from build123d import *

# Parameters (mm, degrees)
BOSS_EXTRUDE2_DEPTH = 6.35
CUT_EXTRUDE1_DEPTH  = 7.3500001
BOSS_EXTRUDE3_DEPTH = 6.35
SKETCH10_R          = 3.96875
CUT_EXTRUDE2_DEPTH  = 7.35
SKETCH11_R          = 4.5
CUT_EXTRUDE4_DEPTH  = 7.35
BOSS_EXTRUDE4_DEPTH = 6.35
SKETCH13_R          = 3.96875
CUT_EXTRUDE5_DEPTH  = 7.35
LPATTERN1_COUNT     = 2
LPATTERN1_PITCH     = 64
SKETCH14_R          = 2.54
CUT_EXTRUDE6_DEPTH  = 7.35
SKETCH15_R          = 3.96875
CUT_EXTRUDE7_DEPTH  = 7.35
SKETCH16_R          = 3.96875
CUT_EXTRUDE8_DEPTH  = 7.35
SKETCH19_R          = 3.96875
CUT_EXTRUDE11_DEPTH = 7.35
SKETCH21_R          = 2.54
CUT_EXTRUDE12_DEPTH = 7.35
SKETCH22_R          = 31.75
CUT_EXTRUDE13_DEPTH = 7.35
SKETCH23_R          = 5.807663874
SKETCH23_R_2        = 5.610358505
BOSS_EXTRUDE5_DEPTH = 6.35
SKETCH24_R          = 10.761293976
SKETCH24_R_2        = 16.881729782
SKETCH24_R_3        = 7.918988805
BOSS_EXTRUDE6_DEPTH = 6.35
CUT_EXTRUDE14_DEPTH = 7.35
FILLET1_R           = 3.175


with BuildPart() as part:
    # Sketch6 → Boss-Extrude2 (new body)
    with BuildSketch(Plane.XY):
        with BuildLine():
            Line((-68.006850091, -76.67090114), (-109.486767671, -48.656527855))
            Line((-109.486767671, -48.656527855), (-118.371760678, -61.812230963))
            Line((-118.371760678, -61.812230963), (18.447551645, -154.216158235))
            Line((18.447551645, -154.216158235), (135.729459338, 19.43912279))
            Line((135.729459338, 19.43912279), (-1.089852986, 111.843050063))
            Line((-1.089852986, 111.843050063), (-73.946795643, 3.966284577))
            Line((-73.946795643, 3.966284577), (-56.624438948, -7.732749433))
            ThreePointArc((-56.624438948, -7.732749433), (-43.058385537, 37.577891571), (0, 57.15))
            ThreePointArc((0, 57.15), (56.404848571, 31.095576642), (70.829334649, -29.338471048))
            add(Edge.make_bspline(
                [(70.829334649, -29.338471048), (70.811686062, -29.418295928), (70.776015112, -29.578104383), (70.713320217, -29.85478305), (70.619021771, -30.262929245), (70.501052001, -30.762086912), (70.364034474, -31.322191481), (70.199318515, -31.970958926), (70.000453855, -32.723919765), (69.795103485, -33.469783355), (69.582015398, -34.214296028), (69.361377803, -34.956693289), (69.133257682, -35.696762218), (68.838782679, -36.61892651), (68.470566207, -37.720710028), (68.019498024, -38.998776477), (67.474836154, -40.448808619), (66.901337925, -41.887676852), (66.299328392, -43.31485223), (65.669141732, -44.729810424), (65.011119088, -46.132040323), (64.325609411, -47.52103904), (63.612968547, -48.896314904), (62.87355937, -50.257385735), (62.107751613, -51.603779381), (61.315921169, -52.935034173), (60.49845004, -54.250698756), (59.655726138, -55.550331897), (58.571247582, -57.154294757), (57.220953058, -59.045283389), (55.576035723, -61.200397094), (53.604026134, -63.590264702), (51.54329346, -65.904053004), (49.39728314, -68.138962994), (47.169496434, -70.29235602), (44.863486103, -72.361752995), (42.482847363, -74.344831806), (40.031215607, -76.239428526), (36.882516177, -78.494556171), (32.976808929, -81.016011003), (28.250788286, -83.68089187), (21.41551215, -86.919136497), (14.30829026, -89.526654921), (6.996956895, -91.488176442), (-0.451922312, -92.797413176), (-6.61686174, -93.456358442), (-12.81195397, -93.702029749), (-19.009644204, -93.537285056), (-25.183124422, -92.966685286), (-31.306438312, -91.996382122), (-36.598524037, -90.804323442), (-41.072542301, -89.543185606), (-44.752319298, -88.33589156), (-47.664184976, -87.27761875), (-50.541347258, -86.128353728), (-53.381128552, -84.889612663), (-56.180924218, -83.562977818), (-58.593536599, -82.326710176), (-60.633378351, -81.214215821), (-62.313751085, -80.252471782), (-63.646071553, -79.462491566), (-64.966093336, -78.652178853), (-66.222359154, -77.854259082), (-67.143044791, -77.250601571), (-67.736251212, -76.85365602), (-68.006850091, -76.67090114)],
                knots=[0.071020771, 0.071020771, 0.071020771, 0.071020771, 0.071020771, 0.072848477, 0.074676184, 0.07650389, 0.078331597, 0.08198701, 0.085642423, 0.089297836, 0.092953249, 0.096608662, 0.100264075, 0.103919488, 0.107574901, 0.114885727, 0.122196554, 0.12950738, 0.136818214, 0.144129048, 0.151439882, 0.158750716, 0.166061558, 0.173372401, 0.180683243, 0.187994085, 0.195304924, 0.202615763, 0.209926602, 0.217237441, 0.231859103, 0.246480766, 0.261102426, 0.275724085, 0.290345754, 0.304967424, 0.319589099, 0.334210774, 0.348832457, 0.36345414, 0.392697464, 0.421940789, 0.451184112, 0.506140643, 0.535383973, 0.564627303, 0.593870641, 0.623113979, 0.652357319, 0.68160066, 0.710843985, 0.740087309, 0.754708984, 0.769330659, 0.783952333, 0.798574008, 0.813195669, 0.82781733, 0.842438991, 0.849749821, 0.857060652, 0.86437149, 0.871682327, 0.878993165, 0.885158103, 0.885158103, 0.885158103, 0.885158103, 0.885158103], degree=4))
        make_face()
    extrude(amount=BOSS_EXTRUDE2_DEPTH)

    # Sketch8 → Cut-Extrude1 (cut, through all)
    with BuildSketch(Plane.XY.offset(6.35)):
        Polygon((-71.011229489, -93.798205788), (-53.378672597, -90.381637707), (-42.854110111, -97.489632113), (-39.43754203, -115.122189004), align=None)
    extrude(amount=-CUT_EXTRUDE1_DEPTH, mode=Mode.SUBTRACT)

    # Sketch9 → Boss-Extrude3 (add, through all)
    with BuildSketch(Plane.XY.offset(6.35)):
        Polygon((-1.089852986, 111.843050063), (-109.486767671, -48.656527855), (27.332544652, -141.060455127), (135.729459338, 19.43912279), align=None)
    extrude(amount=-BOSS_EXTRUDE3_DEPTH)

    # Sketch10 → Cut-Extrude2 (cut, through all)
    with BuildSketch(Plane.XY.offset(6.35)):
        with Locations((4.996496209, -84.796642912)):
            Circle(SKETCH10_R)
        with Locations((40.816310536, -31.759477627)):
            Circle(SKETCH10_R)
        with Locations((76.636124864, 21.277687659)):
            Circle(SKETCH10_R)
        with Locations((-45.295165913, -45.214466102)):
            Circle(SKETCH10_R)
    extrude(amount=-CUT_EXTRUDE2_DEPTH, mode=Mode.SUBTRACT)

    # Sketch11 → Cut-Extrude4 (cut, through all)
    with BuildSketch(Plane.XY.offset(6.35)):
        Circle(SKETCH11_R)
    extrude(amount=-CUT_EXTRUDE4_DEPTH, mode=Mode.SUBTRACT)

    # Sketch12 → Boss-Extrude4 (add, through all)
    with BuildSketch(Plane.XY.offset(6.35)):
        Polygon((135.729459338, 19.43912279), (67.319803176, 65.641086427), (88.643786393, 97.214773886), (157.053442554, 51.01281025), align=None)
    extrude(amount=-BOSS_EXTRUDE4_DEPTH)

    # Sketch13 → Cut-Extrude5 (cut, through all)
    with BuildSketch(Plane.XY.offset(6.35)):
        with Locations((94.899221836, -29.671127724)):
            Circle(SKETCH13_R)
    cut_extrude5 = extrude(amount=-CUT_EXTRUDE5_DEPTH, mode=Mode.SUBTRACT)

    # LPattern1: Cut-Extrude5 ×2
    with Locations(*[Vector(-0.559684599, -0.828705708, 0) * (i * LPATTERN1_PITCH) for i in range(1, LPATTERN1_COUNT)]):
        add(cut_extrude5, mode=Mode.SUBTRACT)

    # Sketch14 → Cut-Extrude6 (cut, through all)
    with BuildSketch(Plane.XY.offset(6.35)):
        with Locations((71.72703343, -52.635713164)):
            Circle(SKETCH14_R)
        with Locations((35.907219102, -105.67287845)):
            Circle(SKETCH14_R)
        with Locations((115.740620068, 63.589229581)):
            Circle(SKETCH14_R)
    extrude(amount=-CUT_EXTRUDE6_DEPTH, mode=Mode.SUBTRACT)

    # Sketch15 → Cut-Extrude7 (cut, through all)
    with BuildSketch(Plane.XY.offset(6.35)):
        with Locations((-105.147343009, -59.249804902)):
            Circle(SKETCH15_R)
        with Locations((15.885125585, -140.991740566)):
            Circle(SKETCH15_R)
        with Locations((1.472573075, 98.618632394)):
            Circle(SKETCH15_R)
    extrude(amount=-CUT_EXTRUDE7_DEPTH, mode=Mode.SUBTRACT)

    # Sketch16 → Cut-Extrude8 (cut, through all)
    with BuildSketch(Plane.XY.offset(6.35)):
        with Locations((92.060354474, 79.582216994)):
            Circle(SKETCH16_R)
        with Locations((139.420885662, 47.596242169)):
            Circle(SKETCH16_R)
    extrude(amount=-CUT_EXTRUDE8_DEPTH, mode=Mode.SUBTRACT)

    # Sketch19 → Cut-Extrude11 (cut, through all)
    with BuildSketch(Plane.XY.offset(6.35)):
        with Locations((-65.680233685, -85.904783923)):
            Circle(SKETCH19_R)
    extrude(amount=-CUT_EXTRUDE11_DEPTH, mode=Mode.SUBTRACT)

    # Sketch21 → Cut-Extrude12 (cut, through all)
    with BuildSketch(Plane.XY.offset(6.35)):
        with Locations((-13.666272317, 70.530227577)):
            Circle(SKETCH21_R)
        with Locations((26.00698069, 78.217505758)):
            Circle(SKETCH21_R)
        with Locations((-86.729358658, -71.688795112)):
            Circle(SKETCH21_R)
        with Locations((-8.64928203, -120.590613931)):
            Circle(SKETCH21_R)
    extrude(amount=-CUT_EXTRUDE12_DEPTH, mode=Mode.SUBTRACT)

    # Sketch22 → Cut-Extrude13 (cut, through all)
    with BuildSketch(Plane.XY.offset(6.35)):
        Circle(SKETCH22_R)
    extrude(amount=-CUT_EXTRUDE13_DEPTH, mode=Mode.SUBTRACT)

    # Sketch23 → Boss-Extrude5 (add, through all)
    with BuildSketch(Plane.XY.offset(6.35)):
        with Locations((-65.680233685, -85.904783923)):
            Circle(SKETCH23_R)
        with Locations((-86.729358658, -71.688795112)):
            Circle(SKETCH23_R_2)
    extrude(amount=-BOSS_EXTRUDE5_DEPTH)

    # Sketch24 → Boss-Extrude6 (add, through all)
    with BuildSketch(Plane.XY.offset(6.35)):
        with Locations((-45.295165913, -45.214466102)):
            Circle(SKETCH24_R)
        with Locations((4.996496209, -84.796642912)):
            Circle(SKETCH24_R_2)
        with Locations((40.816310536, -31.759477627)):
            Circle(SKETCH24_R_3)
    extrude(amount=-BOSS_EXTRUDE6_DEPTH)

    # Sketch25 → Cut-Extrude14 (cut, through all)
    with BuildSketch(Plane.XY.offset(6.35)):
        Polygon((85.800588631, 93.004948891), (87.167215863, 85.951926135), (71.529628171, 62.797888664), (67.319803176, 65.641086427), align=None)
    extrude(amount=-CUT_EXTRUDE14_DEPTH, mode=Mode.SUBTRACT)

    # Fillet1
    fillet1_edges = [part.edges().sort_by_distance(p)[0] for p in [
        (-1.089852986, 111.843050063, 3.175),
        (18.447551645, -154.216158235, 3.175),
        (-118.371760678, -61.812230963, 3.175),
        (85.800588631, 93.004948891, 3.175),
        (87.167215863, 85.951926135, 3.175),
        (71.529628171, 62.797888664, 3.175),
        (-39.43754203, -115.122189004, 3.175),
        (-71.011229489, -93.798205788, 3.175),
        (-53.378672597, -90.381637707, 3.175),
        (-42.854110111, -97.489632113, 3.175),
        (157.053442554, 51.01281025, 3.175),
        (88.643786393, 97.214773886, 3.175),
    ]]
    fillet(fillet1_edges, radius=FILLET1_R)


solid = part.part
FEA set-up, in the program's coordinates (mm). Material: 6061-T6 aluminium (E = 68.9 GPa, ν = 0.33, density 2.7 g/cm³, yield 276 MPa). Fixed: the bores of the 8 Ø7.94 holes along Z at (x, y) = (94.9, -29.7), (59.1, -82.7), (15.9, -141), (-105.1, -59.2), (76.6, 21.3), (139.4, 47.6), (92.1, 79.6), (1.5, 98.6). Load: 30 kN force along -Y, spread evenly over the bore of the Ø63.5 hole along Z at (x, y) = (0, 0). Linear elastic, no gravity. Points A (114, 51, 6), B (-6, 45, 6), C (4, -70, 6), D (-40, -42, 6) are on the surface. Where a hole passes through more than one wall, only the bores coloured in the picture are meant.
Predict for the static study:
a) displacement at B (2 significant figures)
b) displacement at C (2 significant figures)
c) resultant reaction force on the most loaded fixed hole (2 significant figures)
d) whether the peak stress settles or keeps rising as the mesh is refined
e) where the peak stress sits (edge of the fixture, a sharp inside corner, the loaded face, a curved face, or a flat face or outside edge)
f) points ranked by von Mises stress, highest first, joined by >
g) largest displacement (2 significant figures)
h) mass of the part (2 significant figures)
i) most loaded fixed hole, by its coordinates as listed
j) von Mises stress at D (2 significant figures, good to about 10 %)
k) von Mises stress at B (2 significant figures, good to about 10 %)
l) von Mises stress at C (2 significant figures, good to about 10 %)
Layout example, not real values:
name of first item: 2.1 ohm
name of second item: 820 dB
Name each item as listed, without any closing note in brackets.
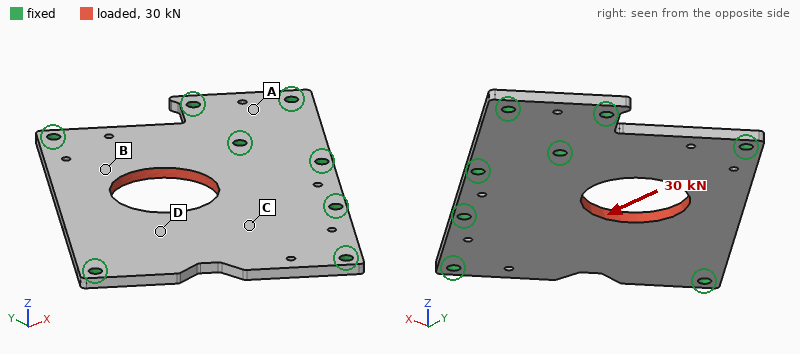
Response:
displacement at B: 33 µm
displacement at C: 29 µm
resultant reaction force on the most loaded fixed hole: 8.6 kN
whether the peak stress settles or keeps rising as the mesh is refined: keeps rising
where the peak stress sits: edge of the fixture
points ranked by von Mises stress, highest first, joined by >: B > C > D > A
largest displacement: 58 µm
mass of the part: 580 g
most loaded fixed hole, by its coordinates as listed: (1.5, 98.6)
von Mises stress at D: 14 MPa
von Mises stress at B: 34 MPa
von Mises stress at C: 26 MPa
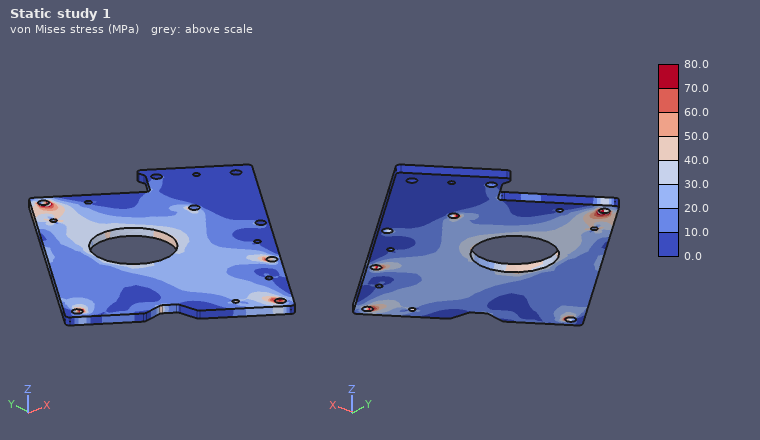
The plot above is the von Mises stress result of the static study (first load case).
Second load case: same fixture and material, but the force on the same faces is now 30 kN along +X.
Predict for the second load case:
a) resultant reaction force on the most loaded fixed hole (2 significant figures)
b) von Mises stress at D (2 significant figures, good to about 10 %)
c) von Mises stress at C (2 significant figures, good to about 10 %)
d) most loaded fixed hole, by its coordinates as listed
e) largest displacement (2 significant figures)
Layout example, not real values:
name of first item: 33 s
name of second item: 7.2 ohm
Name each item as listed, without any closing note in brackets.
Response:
resultant reaction force on the most loaded fixed hole: 8.4 kN
von Mises stress at D: 22 MPa
von Mises stress at C: 14 MPa
most loaded fixed hole, by its coordinates as listed: (76.6, 21.3)
largest displacement: 69 µm
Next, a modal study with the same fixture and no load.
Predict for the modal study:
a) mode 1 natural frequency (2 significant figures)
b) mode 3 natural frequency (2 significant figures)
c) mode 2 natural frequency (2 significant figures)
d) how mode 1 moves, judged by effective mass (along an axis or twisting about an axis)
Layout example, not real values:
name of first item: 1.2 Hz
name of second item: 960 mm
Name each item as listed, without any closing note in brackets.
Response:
mode 1 natural frequency: 960 Hz
mode 3 natural frequency: 2300 Hz
mode 2 natural frequency: 1500 Hz
how mode 1 moves, judged by effective mass: along Z
